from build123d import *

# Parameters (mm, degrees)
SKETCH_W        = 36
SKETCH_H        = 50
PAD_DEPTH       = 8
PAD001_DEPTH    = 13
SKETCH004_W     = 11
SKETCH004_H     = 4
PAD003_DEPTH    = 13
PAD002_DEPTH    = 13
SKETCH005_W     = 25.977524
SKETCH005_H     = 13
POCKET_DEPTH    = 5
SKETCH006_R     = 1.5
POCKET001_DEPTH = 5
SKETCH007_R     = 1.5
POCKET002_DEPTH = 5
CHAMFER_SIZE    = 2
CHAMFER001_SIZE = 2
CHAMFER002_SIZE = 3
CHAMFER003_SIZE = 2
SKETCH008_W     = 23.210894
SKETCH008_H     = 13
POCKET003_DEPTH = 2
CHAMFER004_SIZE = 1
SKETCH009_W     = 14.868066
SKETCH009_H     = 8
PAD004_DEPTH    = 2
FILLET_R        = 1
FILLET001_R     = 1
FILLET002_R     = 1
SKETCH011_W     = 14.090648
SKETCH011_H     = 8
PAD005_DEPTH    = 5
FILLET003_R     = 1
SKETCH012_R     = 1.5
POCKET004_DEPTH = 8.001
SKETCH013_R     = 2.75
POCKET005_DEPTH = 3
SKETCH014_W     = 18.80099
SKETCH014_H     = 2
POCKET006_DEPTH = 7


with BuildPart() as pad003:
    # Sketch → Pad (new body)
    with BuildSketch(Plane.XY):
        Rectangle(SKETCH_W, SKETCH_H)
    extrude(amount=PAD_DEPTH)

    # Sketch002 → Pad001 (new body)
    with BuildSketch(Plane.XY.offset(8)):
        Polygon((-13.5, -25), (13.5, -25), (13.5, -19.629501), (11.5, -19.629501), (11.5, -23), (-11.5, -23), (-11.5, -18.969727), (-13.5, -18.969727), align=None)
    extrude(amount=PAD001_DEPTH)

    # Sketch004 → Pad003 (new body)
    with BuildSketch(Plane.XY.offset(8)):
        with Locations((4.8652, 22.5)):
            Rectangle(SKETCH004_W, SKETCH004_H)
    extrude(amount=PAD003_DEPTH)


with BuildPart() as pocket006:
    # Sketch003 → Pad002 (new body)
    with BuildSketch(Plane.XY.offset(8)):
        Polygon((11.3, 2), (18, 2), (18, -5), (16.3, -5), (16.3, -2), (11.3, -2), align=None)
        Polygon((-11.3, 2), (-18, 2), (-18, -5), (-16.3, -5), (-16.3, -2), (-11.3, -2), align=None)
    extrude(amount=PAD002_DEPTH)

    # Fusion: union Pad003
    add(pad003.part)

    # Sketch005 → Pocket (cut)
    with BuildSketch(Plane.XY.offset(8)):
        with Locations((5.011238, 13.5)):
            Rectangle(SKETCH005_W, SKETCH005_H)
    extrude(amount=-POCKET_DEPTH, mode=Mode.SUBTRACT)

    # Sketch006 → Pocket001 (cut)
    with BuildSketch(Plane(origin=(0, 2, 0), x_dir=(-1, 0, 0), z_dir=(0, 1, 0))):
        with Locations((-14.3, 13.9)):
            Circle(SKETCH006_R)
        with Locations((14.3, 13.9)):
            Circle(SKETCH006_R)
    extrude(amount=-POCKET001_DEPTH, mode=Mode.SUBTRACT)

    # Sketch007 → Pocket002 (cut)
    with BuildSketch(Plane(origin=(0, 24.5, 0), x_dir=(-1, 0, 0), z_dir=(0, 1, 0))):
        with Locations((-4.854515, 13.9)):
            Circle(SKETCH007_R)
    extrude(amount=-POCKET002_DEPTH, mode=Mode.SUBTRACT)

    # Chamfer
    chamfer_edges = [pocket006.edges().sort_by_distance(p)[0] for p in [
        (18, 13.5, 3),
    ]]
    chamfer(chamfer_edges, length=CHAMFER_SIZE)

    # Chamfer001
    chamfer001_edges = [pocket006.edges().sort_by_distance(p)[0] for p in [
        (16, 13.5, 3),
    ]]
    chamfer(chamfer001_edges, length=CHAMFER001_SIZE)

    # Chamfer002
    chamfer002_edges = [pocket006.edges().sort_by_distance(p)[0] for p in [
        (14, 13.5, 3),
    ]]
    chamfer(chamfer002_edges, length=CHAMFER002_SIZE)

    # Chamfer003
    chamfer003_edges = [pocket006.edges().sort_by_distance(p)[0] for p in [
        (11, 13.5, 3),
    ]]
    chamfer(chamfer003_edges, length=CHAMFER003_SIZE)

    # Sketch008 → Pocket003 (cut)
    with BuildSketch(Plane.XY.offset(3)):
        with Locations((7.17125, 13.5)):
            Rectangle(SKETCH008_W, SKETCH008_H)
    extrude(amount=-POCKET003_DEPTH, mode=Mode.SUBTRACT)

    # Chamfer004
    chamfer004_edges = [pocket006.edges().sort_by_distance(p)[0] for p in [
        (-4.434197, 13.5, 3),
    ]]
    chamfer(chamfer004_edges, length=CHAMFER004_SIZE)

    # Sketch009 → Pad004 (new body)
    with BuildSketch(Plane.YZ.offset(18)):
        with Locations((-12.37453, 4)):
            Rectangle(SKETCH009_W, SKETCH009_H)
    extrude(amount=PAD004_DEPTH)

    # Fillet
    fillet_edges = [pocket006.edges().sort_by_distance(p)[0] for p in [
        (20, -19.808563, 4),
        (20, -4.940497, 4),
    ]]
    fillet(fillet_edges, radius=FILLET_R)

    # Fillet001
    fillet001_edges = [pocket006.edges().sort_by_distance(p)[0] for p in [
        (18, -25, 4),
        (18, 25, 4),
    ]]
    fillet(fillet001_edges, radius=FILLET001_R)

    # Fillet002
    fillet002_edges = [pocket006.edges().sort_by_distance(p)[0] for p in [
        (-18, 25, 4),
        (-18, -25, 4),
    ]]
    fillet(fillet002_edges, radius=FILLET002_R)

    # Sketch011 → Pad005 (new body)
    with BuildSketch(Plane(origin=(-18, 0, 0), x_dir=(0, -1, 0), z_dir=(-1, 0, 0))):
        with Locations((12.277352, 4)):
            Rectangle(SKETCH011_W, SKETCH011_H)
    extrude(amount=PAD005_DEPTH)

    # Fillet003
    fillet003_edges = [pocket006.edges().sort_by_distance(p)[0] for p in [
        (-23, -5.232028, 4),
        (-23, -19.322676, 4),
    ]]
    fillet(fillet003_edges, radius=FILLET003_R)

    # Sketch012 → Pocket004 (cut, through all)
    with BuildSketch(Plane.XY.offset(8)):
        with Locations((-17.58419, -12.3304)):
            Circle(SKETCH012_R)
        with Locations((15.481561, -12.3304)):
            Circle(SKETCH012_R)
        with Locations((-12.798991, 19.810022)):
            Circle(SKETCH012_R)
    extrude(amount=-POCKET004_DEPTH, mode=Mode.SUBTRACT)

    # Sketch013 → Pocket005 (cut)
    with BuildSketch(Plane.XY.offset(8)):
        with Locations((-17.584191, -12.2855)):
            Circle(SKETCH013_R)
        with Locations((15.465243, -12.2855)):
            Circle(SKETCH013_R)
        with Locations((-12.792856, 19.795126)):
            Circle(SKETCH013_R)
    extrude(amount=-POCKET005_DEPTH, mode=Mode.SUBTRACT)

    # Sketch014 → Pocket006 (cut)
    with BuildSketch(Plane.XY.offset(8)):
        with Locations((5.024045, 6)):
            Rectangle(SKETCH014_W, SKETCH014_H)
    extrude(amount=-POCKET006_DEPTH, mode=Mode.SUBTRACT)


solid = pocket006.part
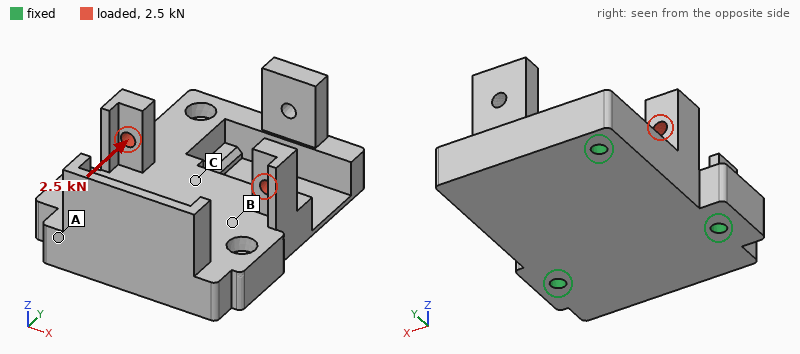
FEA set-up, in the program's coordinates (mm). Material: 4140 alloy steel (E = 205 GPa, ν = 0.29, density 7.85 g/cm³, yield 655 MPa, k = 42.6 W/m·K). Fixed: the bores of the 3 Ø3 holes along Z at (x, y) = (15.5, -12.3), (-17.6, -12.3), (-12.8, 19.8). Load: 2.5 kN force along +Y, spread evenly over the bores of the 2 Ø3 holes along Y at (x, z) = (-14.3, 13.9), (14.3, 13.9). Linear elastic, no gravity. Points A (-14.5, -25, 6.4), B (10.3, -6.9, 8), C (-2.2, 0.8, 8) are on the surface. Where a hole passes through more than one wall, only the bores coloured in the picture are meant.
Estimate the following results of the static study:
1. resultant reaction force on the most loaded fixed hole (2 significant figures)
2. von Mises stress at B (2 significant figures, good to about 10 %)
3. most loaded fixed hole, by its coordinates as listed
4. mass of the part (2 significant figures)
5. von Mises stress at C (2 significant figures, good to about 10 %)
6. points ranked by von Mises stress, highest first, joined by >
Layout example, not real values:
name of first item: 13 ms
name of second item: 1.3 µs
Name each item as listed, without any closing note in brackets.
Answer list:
resultant reaction force on the most loaded fixed hole: 1.2 kN
von Mises stress at B: 57 MPa
most loaded fixed hole, by its coordinates as listed: (15.5, -12.3)
mass of the part: 110 g
von Mises stress at C: 35 MPa
points ranked by von Mises stress, highest first, joined by >: B > C > A
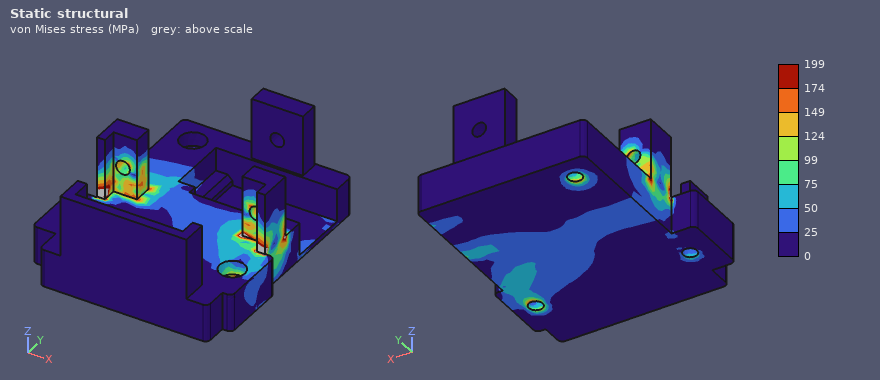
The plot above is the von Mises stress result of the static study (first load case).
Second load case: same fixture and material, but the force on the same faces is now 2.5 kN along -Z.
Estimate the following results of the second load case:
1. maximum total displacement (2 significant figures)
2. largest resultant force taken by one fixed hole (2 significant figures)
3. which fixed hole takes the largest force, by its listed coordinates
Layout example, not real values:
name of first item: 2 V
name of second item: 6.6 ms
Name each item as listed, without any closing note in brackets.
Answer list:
maximum total displacement: 27 µm
largest resultant force taken by one fixed hole: 1.2 kN
which fixed hole takes the largest force, by its listed coordinates: (15.5, -12.3)
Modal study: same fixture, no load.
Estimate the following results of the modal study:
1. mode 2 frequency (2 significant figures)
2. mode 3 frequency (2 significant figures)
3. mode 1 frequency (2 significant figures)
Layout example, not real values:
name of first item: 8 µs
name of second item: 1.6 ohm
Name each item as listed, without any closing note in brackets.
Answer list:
mode 2 frequency: 6100 Hz
mode 3 frequency: 9600 Hz
mode 1 frequency: 5100 Hz
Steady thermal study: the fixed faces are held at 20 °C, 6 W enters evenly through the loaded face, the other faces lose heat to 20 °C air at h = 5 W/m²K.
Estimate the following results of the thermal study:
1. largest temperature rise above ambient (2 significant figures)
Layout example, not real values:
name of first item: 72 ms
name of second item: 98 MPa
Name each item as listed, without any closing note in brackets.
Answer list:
largest temperature rise above ambient: 28 K
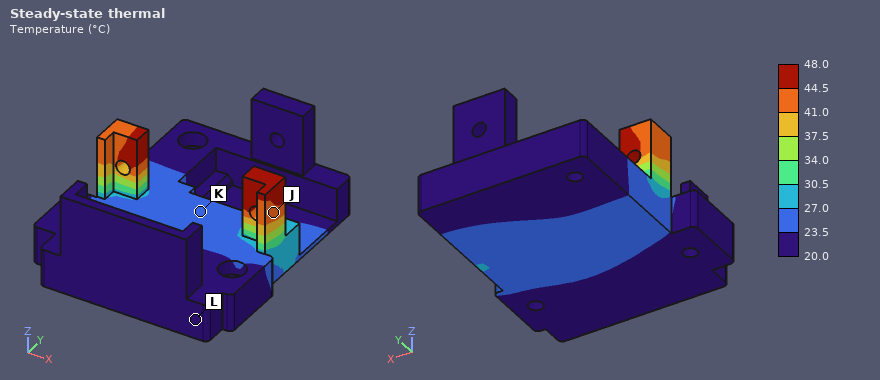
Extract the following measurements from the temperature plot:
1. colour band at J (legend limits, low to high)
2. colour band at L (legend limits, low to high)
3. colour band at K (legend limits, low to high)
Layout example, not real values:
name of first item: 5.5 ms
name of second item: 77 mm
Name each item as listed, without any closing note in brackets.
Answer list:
colour band at J: 41.0 to 44.5 °C
colour band at L: 20.0 to 23.5 °C
colour band at K: 23.5 to 27.0 °C
